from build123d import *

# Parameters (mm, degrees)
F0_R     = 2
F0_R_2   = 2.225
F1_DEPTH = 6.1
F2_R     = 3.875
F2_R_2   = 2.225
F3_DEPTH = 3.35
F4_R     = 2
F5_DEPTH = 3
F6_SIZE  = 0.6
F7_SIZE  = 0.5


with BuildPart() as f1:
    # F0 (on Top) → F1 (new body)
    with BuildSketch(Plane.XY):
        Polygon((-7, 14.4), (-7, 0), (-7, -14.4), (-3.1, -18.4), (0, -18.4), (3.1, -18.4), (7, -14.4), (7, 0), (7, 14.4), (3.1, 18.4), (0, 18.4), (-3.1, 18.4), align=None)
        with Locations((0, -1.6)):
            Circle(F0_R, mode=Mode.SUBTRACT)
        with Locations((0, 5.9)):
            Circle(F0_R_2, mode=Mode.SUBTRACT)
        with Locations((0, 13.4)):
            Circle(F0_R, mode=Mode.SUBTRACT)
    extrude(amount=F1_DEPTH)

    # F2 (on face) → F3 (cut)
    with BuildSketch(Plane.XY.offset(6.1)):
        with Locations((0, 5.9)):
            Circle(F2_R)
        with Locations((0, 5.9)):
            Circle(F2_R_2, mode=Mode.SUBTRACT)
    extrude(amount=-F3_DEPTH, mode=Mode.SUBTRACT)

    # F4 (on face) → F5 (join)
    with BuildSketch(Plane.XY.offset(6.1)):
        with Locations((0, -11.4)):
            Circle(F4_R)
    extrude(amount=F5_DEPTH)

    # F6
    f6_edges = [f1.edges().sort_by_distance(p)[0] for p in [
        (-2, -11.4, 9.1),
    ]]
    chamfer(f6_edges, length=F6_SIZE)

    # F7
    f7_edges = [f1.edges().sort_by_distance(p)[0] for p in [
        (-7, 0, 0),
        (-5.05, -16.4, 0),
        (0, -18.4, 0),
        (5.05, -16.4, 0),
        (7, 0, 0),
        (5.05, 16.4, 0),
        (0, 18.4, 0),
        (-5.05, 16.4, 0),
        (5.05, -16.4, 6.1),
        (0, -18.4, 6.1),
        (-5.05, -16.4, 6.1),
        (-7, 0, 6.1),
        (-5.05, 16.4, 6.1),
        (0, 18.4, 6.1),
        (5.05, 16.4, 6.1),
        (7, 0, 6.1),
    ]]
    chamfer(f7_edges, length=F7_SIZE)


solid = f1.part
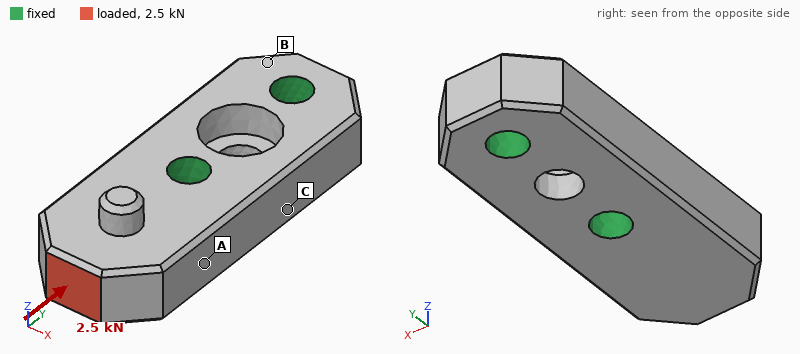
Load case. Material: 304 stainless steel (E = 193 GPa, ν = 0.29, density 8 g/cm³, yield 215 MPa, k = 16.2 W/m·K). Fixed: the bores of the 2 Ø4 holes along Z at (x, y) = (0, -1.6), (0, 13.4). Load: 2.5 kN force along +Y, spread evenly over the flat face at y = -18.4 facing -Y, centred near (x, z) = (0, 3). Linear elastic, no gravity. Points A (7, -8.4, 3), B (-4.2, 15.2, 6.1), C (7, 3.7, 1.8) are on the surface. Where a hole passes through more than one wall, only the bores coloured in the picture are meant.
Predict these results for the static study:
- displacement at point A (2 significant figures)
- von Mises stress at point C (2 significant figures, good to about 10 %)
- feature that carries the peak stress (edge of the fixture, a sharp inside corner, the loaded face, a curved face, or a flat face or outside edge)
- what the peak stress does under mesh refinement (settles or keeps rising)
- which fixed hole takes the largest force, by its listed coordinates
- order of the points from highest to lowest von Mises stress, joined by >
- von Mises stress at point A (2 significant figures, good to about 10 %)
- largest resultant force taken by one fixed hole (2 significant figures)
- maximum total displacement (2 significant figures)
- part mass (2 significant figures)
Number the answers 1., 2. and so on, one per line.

1. 1.3 µm
2. 11 MPa
3. edge of the fixture
4. keeps rising
5. (0, -1.6)
6. A > C > B
7. 19 MPa
8. 2.2 kN
9. 3.9 µm
10. 21 g
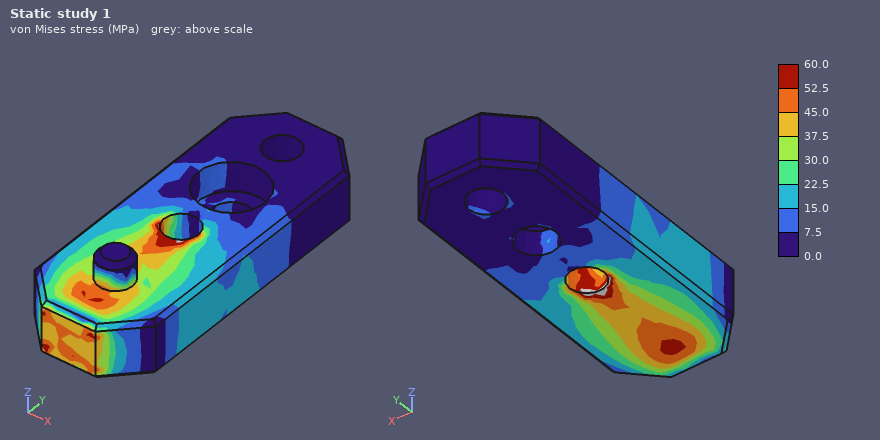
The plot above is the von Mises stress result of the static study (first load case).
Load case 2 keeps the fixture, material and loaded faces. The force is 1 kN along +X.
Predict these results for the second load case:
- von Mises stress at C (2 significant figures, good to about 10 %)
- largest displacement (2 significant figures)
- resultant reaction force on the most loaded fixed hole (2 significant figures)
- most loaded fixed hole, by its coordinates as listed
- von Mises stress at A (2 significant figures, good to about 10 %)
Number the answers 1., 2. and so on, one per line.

1. 40 MPa
2. 14 µm
3. 1.4 kN
4. (0, -1.6)
5. 52 MPa
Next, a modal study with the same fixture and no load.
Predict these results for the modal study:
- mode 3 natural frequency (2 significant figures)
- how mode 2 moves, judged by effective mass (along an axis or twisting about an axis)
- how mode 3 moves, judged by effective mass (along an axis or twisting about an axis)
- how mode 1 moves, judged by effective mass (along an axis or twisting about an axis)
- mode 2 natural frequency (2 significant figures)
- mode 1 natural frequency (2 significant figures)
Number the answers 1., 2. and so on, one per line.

1. 36 kHz
2. along X
3. twisting about Y
4. along Z
5. 24 kHz
6. 18 kHz
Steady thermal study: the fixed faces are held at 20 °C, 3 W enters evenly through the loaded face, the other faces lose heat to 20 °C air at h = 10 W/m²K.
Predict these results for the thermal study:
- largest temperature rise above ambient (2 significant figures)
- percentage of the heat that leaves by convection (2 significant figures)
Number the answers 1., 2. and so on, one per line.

1. 44 K
2. 4.1 %
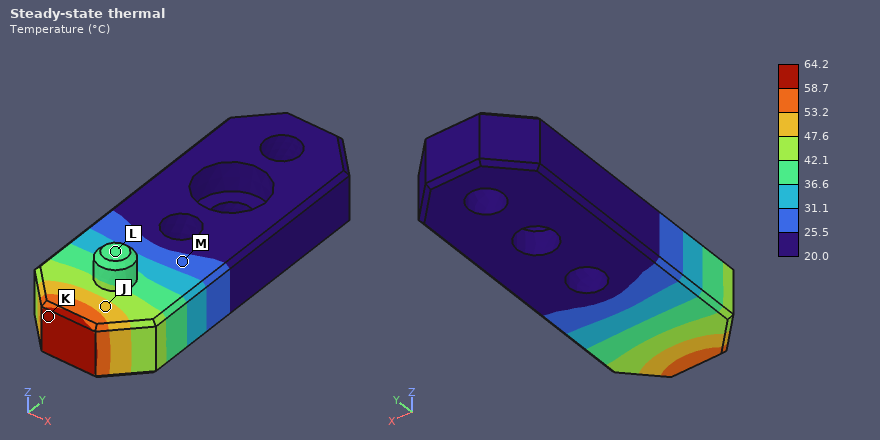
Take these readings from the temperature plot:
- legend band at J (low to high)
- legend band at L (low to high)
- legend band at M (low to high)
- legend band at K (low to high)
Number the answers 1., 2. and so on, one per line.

1. 47.6 to 53.2 °C
2. 36.6 to 42.1 °C
3. 25.5 to 31.1 °C
4. 58.7 to 64.2 °C
